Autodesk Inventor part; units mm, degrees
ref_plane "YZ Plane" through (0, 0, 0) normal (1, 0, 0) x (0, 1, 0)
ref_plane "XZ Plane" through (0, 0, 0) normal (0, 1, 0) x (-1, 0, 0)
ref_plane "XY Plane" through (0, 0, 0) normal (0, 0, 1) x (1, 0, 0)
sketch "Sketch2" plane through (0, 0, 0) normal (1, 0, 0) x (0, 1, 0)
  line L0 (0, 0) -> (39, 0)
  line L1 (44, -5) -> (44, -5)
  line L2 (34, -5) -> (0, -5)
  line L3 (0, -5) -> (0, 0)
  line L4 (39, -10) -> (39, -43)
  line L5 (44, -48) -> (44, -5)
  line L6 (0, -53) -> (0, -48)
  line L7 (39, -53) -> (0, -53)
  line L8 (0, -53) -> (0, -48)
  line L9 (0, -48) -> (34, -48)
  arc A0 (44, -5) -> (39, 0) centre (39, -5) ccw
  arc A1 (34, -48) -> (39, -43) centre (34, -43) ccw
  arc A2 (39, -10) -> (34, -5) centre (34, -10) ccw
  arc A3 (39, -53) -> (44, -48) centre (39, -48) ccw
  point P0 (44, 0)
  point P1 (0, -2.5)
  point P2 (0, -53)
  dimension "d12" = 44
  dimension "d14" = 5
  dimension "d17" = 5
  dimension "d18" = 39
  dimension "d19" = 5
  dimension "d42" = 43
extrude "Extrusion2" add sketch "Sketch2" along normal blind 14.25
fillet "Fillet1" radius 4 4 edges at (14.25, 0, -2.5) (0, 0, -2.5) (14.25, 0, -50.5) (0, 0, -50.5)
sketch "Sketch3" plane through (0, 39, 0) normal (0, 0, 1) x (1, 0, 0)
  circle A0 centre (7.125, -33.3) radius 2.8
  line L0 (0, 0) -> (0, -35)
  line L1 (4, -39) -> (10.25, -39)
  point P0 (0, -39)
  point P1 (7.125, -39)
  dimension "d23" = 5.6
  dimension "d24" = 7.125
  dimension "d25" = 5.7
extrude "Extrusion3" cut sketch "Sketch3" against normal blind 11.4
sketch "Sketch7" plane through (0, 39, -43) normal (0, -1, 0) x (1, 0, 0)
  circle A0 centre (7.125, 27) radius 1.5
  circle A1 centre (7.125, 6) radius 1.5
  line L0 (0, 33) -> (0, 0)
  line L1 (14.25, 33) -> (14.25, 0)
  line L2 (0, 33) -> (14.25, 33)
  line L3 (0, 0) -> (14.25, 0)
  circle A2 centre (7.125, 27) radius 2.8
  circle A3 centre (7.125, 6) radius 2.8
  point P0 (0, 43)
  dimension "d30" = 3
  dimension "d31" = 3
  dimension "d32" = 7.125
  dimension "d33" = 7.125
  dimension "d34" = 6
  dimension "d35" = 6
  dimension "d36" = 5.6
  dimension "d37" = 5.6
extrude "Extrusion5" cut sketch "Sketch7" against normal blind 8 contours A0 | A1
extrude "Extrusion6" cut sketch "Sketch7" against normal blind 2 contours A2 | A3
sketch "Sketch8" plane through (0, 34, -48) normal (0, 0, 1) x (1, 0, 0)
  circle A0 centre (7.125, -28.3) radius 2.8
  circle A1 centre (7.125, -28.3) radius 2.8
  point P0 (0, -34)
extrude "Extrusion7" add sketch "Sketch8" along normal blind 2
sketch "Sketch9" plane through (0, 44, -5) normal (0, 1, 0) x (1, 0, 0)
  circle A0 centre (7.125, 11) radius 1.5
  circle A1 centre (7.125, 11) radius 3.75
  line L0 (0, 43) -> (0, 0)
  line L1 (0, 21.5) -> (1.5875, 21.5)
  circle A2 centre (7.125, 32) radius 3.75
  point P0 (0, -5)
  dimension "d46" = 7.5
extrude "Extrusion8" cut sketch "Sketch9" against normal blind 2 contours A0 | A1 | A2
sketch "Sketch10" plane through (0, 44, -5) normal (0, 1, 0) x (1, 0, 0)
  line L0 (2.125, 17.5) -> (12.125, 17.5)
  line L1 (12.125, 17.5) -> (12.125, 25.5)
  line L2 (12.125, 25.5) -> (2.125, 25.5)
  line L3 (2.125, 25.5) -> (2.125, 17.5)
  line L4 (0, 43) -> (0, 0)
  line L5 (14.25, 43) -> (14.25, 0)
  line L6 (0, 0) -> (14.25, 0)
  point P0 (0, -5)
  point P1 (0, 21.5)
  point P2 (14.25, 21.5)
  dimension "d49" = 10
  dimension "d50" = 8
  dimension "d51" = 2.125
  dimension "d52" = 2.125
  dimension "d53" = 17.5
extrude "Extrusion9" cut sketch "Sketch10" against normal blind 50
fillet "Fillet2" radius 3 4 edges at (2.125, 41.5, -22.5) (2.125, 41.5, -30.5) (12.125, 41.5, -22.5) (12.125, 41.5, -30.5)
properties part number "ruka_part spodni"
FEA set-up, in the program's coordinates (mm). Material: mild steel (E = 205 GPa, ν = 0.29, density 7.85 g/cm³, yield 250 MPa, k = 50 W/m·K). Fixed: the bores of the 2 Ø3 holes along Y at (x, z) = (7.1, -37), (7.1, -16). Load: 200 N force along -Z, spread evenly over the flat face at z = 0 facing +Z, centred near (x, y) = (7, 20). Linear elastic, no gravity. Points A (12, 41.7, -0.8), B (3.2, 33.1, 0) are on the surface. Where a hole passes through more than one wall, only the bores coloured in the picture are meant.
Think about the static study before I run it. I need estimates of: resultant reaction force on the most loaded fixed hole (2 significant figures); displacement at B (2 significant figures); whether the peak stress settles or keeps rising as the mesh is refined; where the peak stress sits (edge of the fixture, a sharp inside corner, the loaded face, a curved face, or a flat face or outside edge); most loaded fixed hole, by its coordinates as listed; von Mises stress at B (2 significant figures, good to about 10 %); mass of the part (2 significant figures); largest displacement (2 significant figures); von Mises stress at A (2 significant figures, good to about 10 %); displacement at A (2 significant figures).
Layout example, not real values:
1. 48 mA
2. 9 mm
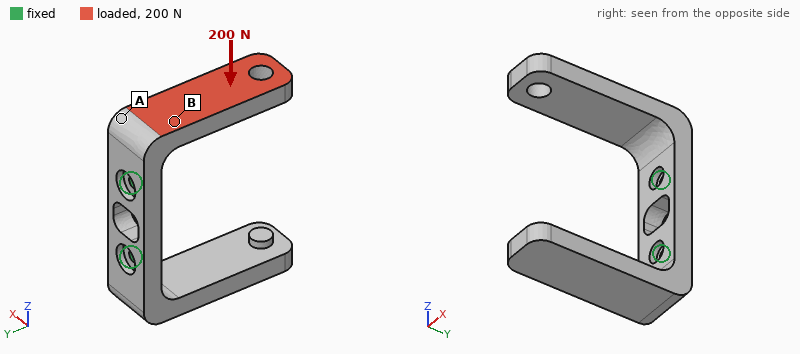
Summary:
1. 220 N
2. 0.057 mm
3. keeps rising
4. edge of the fixture
5. (7.1, -16)
6. 43 MPa
7. 67 g
8. 0.19 mm
9. 16 MPa
10. 0.044 mm
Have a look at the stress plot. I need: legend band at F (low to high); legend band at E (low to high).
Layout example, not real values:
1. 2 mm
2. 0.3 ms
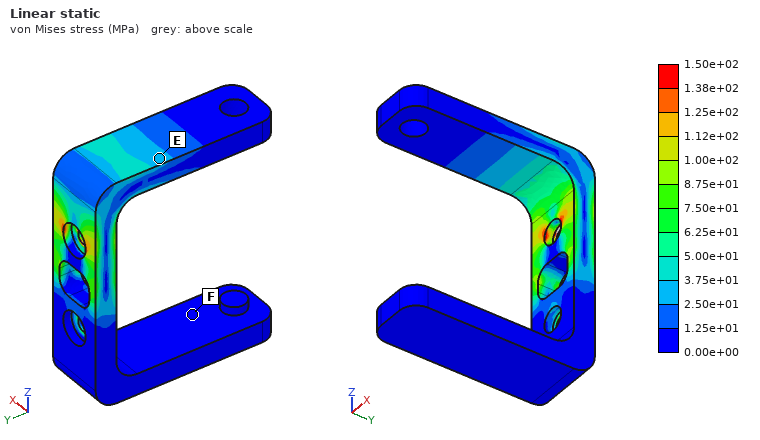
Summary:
1. 0.00e+00 to 1.25e+01 MPa
2. 2.50e+01 to 3.75e+01 MPa
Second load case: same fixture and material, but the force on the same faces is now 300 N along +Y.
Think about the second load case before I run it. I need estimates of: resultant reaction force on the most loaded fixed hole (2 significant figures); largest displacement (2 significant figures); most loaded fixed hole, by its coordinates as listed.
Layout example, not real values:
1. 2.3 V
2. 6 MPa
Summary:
1. 490 N
2. 0.16 mm
3. (7.1, -16)
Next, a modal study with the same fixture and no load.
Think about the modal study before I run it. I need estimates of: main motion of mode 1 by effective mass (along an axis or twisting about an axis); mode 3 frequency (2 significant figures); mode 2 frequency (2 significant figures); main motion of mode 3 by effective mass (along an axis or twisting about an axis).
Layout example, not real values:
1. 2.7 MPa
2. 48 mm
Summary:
1. along X
2. 1400 Hz
3. 1200 Hz
4. along Z
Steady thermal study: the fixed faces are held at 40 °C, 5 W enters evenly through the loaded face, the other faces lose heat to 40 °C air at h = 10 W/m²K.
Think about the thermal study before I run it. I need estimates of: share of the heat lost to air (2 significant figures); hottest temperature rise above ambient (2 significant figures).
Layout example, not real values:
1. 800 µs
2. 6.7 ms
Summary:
1. 12 %
2. 49 K
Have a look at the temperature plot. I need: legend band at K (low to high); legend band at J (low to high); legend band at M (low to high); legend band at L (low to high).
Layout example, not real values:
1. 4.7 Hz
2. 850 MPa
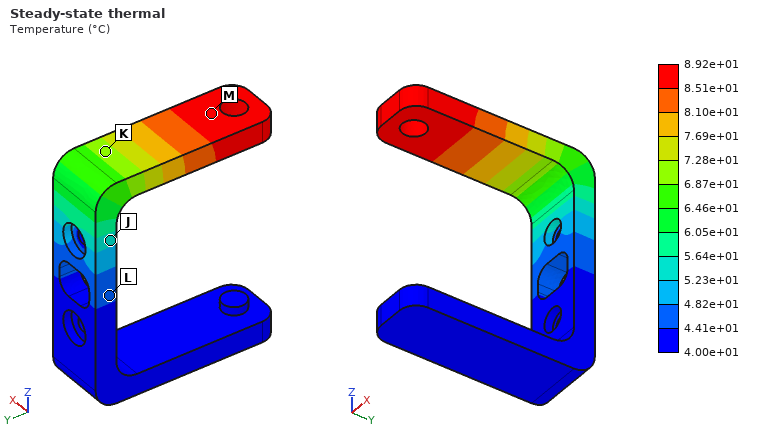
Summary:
1. 6.87e+01 to 7.28e+01 °C
2. 5.23e+01 to 5.64e+01 °C
3. 8.51e+01 to 8.92e+01 °C
4. 4.41e+01 to 4.82e+01 °C
